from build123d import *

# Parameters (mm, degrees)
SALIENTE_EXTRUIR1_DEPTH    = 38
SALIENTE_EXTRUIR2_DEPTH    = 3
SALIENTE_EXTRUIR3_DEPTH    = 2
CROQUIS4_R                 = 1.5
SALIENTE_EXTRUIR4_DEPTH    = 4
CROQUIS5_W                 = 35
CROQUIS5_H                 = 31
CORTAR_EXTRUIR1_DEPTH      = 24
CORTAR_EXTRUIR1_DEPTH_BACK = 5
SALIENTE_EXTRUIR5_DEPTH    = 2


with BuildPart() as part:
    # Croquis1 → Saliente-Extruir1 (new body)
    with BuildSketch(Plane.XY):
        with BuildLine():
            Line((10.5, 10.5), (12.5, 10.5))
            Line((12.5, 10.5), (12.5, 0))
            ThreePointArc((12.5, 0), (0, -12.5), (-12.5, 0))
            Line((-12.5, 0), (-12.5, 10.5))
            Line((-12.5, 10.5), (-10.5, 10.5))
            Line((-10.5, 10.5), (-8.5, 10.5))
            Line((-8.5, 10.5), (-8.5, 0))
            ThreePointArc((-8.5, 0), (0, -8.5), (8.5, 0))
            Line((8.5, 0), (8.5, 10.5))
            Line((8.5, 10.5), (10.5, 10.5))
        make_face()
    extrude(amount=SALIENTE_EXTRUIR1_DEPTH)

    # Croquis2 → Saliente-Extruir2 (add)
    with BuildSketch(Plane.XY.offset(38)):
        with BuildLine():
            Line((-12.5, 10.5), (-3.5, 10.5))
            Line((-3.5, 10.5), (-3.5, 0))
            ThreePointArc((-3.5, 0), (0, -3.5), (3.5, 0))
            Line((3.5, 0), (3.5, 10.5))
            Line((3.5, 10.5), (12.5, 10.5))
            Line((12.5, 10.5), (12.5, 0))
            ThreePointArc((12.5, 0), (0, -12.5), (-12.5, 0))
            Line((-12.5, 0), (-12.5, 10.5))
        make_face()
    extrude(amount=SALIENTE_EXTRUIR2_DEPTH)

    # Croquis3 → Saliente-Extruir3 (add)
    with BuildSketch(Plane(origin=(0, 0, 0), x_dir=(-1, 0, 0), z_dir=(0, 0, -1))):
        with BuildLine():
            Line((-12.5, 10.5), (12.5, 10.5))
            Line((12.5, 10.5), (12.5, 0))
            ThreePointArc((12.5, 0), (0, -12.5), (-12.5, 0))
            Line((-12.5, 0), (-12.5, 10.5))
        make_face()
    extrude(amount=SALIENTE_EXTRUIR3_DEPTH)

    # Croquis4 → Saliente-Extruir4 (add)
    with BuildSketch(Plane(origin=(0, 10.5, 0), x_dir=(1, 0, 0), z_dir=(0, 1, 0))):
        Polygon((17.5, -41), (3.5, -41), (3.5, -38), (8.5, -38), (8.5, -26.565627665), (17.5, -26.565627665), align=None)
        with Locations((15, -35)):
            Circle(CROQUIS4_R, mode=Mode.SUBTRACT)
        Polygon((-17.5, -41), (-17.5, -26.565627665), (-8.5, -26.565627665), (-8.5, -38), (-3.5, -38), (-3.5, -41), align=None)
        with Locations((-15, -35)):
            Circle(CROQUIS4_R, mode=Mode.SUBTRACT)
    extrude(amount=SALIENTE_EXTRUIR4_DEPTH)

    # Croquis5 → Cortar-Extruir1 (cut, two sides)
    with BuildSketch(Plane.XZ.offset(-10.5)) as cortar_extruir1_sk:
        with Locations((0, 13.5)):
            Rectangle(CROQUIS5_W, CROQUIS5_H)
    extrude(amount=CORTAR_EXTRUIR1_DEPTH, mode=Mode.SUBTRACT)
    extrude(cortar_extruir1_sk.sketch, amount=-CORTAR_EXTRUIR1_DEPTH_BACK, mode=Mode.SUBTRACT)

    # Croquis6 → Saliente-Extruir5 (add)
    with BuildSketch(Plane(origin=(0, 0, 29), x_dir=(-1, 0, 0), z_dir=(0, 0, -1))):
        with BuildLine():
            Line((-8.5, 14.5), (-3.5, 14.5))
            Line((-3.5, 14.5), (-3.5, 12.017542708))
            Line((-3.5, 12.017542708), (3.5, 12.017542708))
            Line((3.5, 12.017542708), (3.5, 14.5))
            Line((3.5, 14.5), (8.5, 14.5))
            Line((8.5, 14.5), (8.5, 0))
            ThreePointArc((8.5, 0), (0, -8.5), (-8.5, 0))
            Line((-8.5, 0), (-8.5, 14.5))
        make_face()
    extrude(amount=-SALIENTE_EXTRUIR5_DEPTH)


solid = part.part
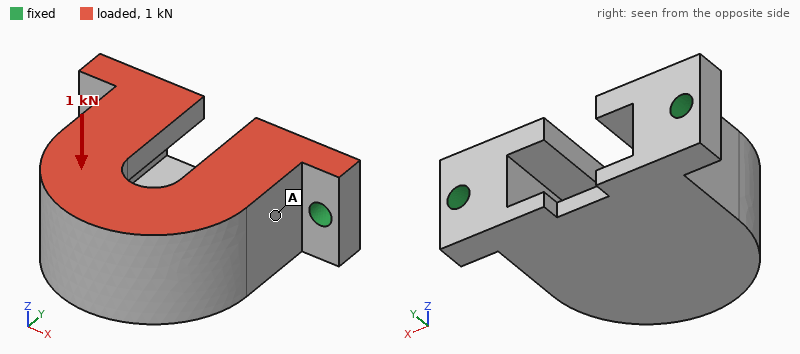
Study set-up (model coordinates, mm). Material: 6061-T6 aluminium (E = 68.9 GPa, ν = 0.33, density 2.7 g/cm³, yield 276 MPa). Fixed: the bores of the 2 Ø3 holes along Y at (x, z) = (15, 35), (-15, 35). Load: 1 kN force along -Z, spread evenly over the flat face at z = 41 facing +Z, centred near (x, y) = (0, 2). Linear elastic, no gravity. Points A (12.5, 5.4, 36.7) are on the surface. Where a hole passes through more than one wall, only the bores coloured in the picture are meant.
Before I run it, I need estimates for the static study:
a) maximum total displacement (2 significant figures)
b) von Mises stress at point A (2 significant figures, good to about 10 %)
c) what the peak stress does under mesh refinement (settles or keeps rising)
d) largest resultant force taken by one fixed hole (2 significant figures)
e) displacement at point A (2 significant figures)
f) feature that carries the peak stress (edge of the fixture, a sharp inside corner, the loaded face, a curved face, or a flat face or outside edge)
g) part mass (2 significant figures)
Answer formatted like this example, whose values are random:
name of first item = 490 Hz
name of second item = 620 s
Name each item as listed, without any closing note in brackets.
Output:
maximum total displacement = 0.10 mm
von Mises stress at point A = 24 MPa
what the peak stress does under mesh refinement = keeps rising
largest resultant force taken by one fixed hole = 510 N
displacement at point A = 0.029 mm
feature that carries the peak stress = edge of the fixture
part mass = 13 g
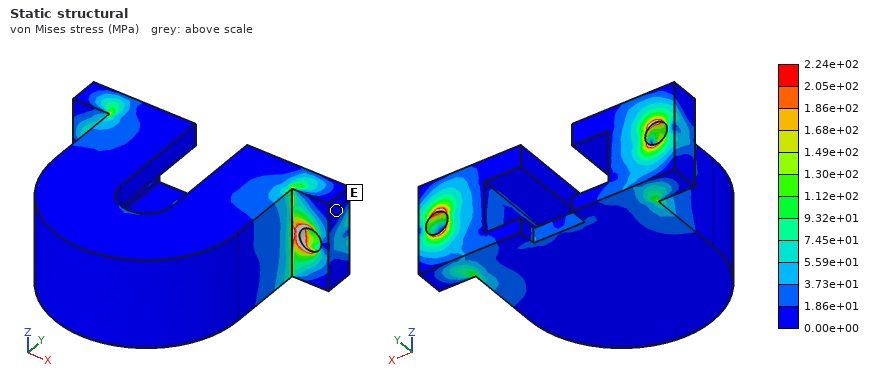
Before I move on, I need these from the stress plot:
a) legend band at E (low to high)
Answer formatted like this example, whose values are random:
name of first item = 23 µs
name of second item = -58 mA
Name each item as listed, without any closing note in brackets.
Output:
legend band at E = 0.00e+00 to 1.86e+01 MPa
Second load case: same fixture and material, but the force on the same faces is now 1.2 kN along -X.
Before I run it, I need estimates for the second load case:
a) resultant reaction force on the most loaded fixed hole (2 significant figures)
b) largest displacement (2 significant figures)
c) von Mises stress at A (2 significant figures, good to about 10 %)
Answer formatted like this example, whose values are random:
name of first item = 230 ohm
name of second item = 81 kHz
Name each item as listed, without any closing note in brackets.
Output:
resultant reaction force on the most loaded fixed hole = 750 N
largest displacement = 28 µm
von Mises stress at A = 21 MPa
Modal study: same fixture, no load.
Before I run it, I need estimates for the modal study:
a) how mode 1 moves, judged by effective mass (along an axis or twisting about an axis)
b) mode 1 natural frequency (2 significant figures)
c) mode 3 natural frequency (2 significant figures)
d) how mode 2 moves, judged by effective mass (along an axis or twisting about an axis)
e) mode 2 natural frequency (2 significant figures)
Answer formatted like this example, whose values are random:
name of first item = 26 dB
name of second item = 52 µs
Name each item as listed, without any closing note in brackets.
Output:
how mode 1 moves, judged by effective mass = along Z
mode 1 natural frequency = 5200 Hz
mode 3 natural frequency = 20 kHz
how mode 2 moves, judged by effective mass = along X
mode 2 natural frequency = 14 kHz
